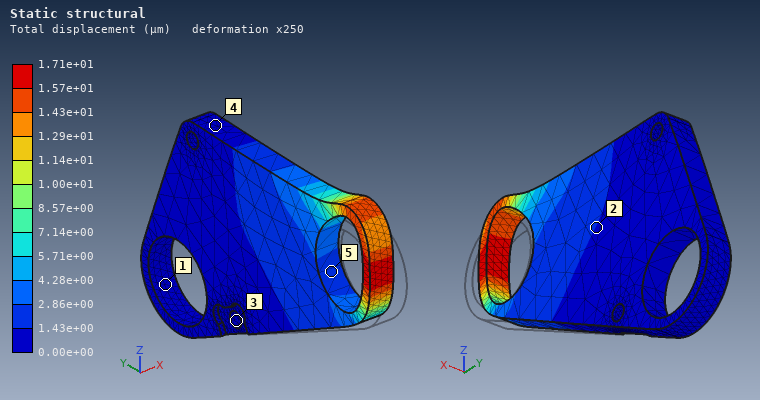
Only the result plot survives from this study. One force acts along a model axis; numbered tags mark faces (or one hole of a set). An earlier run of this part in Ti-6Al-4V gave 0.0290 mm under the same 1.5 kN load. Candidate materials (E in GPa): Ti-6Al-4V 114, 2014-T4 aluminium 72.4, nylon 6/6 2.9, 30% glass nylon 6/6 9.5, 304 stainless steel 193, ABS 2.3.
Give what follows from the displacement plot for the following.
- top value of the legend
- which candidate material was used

1.71e+01 µm
304 stainless steel
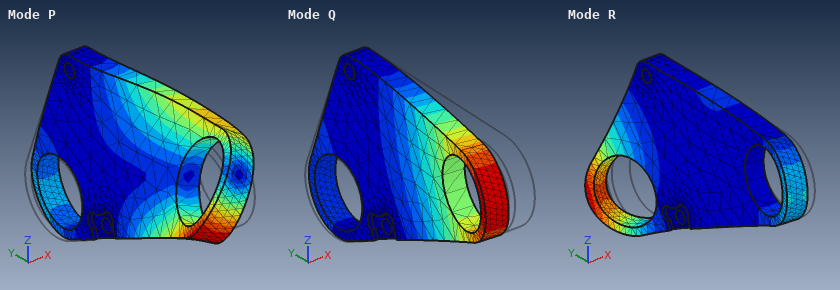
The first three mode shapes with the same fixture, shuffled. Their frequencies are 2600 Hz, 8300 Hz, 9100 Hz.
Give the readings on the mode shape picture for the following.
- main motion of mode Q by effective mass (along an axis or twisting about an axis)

along X
